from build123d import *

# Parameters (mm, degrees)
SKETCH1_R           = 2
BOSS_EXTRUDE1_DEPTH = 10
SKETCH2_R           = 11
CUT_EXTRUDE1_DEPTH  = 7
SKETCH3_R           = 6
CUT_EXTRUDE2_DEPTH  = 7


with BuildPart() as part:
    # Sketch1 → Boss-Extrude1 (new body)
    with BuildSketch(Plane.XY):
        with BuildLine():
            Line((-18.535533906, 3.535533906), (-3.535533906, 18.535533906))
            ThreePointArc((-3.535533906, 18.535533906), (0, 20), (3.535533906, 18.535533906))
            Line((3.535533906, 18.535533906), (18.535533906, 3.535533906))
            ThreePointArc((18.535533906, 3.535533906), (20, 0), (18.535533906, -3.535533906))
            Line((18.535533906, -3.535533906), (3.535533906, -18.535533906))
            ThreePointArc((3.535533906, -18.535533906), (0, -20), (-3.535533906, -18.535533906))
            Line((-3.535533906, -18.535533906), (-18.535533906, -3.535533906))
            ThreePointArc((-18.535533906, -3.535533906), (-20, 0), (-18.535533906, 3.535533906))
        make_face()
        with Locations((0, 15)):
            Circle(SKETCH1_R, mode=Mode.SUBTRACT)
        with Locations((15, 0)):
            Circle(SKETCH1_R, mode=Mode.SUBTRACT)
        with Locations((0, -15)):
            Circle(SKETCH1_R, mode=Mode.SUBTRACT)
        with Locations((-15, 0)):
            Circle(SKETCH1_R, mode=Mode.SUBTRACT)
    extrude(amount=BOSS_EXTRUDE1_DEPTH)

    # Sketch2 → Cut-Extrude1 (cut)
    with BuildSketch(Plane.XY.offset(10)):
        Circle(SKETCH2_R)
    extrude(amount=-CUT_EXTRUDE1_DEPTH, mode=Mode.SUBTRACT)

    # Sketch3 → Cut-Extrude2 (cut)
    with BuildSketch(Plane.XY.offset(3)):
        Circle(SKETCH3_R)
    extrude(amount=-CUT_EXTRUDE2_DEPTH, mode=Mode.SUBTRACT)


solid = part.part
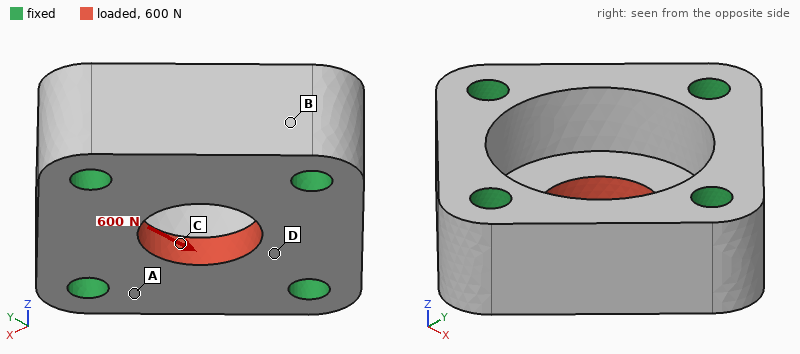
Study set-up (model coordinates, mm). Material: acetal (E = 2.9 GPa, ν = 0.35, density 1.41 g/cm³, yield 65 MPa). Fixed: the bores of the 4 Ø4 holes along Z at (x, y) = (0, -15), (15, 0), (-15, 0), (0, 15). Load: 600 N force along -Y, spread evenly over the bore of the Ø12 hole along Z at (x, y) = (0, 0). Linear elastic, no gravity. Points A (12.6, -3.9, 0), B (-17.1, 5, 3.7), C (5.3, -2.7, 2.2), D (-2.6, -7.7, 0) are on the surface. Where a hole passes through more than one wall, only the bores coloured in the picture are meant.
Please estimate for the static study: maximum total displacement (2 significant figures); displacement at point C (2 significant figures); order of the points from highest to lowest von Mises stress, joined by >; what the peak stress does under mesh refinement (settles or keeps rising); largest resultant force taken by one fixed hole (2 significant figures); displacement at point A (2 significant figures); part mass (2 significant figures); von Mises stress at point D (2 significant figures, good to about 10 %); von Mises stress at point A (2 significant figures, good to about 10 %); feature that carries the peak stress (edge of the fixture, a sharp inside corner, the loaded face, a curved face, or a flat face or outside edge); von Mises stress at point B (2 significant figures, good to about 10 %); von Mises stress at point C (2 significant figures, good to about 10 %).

24 µm
23 µm
C > D > A > B
keeps rising
190 N
5.7 µm
8.5 g
6.4 MPa
2.9 MPa
edge of the fixture
1.2 MPa
8.8 MPa
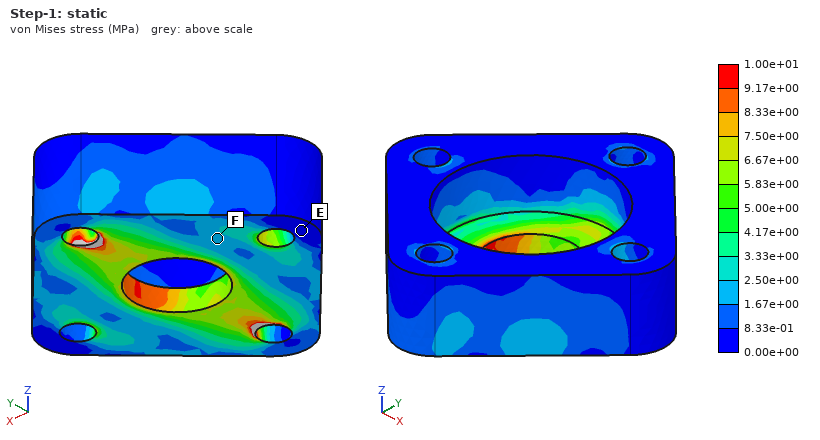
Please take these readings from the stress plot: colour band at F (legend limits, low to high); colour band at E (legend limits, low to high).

1.67e+00 to 2.50e+00 MPa
0.00e+00 to 8.33e-01 MPa
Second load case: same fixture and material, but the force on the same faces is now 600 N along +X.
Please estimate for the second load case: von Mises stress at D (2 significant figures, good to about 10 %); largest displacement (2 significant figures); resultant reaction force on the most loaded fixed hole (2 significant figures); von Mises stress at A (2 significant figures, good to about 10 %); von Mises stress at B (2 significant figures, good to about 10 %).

2.8 MPa
24 µm
190 N
4.3 MPa
2.0 MPa
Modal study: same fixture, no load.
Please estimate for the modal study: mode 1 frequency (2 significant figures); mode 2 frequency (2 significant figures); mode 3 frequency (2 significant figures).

16 kHz
17 kHz
18 kHz
